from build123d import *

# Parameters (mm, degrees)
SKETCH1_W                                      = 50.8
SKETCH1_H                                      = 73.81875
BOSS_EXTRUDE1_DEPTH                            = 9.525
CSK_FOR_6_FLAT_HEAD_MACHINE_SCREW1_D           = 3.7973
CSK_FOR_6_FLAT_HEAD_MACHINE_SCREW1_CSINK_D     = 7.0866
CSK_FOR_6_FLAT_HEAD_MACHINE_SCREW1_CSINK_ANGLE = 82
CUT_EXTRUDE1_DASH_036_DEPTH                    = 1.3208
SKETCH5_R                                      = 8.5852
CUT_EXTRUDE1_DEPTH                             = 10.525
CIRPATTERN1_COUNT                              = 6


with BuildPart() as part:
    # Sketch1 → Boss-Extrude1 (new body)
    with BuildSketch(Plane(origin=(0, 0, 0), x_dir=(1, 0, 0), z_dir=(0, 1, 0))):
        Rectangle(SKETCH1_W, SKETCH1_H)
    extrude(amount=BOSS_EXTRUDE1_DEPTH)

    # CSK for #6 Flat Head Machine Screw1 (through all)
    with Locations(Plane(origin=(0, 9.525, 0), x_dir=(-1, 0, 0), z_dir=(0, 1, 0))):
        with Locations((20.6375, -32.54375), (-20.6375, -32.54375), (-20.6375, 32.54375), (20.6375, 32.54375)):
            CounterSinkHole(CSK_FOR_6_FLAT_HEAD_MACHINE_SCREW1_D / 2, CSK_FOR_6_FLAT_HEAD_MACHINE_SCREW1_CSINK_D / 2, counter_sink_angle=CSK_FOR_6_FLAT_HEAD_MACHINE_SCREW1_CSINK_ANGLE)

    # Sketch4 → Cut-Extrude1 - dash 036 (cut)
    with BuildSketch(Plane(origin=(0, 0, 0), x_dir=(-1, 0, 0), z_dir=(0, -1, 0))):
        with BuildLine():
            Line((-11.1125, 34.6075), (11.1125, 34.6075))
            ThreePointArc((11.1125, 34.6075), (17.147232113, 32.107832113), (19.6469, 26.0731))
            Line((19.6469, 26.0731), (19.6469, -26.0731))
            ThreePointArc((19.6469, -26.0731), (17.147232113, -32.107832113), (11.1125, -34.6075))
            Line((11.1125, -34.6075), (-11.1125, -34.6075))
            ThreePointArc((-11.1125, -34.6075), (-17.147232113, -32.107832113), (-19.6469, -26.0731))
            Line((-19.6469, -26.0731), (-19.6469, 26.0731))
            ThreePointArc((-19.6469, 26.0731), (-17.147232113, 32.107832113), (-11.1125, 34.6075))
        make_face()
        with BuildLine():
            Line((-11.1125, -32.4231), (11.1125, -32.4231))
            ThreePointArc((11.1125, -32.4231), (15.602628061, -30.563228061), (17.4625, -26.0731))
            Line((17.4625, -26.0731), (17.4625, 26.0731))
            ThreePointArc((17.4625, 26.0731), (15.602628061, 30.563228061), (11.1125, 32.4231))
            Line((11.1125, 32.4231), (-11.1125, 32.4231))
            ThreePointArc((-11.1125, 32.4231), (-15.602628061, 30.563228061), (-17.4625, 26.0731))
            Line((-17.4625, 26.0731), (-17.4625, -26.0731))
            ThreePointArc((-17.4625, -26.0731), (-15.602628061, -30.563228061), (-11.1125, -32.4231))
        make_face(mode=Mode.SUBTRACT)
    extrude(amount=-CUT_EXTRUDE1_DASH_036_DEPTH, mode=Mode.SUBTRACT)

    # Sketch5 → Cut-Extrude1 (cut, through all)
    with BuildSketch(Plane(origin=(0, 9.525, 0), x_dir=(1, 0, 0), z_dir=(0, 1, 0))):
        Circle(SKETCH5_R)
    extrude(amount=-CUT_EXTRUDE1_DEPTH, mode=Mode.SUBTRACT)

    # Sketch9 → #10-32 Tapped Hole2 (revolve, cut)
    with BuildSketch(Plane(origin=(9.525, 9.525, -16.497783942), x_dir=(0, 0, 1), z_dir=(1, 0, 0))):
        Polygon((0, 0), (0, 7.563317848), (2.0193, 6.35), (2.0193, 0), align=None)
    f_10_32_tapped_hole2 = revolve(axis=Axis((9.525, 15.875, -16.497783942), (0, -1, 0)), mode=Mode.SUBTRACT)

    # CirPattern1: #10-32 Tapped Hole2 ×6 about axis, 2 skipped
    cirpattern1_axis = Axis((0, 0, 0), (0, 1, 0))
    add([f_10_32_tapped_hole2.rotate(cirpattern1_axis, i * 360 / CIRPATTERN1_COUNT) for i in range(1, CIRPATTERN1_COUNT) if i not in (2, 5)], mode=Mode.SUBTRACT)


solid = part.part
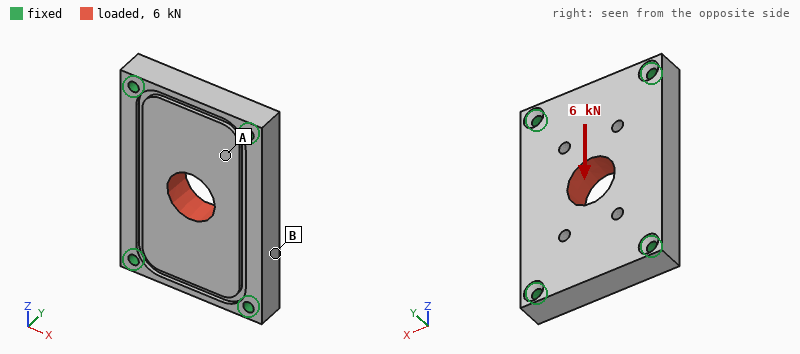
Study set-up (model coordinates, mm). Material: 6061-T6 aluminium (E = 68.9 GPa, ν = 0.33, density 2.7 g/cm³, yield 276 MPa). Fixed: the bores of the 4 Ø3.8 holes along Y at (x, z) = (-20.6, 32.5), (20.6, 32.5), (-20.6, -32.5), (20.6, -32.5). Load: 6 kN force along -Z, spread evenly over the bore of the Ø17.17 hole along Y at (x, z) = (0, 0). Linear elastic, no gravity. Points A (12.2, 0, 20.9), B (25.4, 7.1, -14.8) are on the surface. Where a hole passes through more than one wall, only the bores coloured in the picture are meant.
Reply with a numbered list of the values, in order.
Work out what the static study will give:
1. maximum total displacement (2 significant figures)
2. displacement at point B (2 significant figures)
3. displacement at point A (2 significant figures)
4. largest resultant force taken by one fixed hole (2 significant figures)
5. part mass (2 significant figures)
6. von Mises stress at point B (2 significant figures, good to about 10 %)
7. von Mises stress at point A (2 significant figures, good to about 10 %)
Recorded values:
1. 6.2 µm
2. 2.6 µm
3. 3.3 µm
4. 1.6 kN
5. 87 g
6. 4.3 MPa
7. 10 MPa
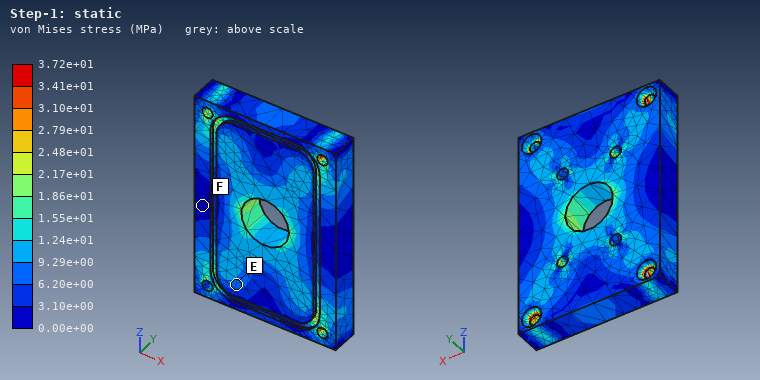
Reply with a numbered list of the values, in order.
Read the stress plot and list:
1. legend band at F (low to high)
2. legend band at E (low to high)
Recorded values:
1. 0.00e+00 to 3.10e+00 MPa
2. 6.20e+00 to 9.29e+00 MPa
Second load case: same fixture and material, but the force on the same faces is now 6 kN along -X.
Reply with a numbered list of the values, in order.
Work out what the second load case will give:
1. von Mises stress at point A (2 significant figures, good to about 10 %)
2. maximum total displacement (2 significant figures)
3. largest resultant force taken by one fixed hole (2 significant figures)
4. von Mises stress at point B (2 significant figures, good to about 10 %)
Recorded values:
1. 14 MPa
2. 12 µm
3. 1.9 kN
4. 5.0 MPa
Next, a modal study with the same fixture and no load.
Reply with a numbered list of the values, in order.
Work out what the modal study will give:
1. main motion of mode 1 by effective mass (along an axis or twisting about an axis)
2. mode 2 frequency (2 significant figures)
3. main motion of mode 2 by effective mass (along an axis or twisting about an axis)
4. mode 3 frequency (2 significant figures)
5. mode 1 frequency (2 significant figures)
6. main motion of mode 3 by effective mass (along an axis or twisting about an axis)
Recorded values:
1. along Y
2. 12 kHz
3. twisting about Z
4. 17 kHz
5. 7600 Hz
6. twisting about X
